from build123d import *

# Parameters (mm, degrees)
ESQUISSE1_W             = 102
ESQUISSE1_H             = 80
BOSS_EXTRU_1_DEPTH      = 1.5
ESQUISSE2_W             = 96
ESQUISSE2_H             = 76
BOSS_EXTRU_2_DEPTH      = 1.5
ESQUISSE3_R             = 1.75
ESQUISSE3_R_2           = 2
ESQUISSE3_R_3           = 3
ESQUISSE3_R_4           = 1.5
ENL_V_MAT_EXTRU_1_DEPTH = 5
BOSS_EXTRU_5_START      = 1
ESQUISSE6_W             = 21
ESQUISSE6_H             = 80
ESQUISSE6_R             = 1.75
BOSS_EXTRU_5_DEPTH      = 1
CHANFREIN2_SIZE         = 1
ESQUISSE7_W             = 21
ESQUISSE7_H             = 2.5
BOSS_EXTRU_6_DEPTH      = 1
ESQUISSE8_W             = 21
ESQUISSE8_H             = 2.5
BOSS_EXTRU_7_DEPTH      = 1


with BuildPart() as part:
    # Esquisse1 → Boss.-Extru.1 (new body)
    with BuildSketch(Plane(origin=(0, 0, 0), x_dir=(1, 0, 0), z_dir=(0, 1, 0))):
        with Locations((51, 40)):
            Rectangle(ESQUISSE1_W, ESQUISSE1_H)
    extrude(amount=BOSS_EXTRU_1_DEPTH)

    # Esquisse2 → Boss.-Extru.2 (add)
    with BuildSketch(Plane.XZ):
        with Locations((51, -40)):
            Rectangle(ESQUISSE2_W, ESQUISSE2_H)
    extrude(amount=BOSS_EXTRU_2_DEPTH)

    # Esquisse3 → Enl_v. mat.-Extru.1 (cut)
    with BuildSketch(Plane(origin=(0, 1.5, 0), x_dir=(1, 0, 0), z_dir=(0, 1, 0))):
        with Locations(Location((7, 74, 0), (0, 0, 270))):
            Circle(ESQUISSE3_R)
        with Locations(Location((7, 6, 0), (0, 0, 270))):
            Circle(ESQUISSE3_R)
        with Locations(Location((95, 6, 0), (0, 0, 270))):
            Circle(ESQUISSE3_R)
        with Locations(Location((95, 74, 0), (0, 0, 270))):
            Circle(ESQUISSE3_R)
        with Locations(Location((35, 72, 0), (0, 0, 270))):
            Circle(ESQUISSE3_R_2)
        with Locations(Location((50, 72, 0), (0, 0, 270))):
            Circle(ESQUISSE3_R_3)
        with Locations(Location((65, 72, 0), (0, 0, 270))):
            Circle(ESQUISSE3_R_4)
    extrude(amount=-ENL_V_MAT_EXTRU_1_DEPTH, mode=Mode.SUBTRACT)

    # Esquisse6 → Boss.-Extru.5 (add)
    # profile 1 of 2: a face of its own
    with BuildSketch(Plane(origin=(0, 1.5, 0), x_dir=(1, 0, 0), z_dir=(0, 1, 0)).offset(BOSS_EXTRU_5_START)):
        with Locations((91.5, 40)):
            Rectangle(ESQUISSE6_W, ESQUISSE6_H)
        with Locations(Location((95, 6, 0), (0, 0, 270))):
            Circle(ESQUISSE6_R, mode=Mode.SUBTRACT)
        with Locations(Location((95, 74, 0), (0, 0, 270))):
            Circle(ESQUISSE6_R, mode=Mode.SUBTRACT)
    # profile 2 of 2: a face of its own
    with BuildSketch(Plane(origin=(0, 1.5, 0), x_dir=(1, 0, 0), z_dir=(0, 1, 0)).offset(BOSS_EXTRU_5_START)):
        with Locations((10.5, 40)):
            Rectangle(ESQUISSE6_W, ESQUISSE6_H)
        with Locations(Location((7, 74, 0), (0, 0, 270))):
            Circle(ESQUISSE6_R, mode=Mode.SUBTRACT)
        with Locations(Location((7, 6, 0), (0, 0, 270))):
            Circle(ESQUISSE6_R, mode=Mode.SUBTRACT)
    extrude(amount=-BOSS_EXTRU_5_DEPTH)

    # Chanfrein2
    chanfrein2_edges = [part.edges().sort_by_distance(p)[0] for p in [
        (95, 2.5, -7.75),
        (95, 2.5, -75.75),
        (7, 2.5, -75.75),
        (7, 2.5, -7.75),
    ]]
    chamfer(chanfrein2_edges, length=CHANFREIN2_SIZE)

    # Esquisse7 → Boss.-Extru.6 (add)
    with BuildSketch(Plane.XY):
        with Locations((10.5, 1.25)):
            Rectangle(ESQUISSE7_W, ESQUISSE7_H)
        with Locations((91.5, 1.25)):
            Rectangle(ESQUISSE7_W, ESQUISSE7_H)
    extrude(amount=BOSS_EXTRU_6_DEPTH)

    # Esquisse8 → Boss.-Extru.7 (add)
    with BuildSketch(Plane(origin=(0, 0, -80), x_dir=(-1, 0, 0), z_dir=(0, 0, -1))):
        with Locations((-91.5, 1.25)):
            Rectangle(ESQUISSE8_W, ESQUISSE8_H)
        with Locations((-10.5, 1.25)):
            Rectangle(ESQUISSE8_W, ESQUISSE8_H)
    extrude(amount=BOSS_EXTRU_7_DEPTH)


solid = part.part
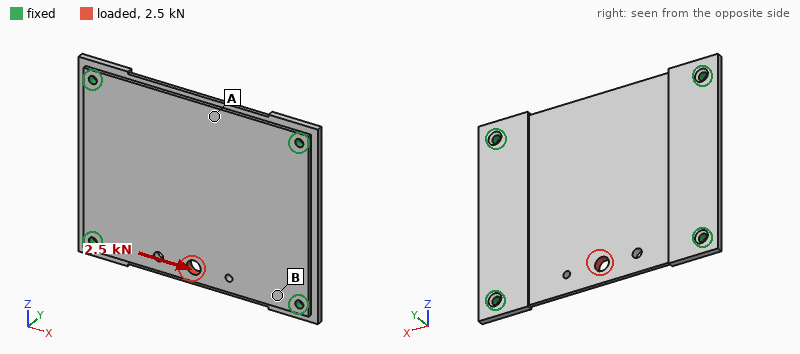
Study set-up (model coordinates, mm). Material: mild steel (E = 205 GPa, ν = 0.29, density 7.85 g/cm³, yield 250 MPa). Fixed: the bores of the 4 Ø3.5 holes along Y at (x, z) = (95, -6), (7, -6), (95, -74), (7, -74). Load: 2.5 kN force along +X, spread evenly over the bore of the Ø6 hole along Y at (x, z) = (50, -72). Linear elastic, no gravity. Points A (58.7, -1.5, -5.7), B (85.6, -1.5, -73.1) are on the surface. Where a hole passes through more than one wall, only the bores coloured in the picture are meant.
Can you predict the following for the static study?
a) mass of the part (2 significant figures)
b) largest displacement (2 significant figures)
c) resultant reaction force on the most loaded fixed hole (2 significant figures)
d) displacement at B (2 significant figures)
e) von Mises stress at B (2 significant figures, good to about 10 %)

210 g
5.7 µm
970 N
1.2 µm
24 MPa
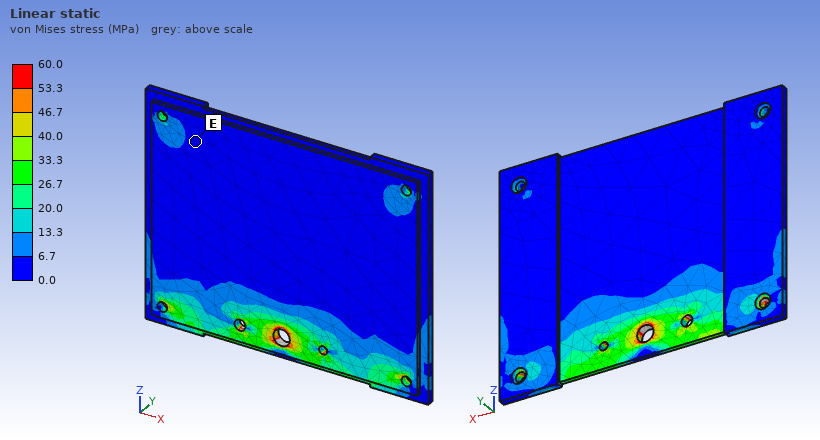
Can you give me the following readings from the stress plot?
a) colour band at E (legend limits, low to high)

0.0 to 6.7 MPa
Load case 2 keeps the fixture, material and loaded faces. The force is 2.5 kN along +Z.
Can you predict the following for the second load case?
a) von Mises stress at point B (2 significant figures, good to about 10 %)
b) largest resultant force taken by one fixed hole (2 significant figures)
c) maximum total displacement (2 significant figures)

8.4 MPa
770 N
9.2 µm
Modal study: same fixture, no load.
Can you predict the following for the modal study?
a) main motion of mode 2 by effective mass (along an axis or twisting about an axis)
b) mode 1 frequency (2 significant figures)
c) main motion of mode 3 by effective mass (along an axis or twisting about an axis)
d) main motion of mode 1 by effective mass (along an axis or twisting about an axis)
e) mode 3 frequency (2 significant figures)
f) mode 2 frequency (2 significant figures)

twisting about X
1800 Hz
twisting about Z
along Y
3700 Hz
2900 Hz
